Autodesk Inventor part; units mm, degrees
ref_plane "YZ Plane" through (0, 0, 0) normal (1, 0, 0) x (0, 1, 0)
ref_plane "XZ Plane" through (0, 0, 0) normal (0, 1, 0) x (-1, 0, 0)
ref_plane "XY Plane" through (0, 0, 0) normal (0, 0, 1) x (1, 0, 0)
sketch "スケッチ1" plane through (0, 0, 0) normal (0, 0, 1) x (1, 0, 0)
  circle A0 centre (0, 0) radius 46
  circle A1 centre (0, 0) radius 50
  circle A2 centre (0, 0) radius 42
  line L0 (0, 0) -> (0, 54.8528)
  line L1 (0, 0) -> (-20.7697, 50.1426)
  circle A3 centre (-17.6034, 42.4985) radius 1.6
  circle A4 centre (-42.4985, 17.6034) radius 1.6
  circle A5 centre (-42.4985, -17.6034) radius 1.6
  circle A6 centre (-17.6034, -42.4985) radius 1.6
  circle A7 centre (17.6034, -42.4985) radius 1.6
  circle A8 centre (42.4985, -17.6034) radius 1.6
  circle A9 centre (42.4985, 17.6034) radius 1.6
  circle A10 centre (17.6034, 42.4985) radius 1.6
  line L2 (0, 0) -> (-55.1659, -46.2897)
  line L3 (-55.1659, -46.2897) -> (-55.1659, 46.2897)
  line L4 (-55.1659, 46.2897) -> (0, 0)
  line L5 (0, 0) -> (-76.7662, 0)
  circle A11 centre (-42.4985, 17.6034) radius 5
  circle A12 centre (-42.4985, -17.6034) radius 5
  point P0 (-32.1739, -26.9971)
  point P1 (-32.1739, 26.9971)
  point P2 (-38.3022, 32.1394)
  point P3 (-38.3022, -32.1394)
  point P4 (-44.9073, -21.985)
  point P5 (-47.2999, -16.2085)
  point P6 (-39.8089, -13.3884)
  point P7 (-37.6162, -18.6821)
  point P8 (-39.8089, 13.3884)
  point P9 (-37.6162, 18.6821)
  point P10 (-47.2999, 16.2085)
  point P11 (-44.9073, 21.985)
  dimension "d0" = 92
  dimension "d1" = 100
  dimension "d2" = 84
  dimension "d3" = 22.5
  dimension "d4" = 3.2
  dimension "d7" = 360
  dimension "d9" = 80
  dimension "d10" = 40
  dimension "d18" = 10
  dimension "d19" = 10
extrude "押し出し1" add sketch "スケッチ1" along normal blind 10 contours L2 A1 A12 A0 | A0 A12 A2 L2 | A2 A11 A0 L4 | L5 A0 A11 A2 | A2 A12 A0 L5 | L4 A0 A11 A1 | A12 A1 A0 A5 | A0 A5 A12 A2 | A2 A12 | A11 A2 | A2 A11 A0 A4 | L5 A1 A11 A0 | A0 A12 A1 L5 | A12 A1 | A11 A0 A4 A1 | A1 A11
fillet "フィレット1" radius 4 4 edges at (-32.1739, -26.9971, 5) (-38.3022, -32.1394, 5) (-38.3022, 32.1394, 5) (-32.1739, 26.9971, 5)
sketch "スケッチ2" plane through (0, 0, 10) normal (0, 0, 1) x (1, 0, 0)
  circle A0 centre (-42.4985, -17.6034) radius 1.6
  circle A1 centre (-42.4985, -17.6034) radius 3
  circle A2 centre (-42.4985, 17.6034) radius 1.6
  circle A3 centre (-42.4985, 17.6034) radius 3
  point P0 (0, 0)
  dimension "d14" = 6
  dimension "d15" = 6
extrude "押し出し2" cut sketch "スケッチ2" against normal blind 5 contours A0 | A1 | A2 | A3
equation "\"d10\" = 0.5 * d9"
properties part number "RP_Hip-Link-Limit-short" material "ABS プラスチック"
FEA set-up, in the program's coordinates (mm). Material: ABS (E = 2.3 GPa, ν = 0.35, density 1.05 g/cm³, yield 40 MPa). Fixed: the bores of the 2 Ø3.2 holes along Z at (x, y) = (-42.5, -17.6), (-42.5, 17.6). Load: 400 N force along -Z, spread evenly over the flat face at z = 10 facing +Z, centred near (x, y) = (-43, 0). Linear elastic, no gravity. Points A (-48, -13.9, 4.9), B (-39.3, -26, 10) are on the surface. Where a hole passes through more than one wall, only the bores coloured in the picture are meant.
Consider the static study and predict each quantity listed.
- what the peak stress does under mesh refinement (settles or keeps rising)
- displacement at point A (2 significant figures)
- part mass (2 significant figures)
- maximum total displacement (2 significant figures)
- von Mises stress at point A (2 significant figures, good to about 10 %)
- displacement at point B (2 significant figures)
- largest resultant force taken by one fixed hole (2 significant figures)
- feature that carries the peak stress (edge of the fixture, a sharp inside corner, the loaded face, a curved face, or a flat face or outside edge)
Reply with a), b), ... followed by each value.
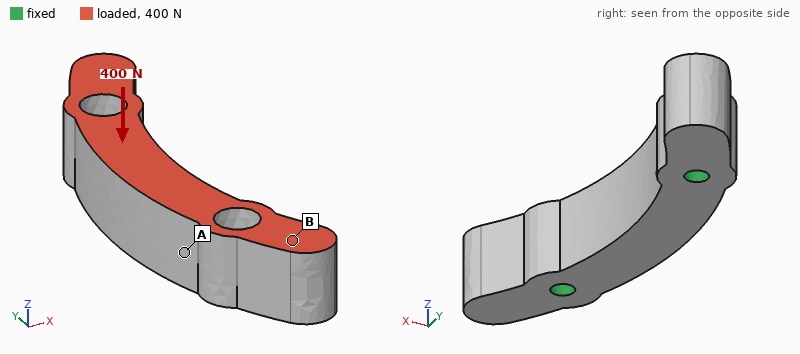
a) keeps rising
b) 23 µm
c) 5.0 g
d) 62 µm
e) 3.7 MPa
f) 31 µm
g) 200 N
h) edge of the fixture
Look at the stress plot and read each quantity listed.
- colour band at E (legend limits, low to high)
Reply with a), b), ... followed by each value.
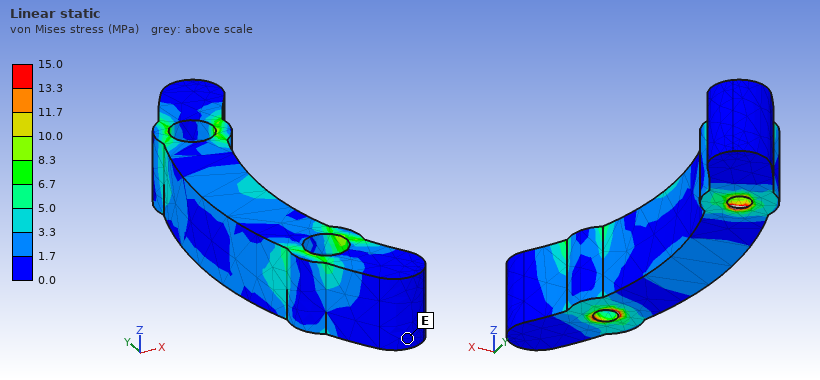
a) 0.0 to 1.7 MPa
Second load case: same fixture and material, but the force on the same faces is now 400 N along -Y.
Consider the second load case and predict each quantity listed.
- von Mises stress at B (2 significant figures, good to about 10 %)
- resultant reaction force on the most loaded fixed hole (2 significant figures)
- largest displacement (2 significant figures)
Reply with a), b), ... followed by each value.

a) 2.3 MPa
b) 210 N
c) 93 µm
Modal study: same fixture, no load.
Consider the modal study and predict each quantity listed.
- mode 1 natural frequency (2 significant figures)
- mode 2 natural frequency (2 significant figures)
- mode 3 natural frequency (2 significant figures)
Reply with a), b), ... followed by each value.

a) 5000 Hz
b) 6100 Hz
c) 6600 Hz
